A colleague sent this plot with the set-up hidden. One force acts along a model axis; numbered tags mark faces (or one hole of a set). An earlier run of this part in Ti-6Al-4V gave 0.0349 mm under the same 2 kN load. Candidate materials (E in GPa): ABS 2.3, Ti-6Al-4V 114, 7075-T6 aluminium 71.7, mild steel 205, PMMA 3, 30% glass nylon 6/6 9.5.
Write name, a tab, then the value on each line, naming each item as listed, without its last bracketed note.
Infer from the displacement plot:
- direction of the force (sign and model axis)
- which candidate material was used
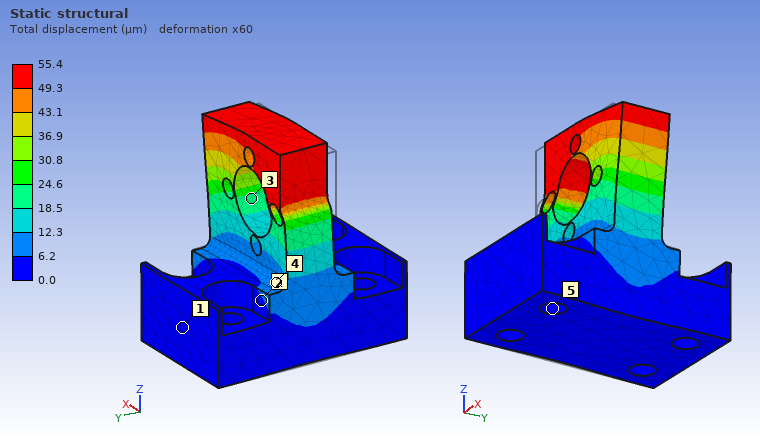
direction of the force	+X
which candidate material was used	7075-T6 aluminium
